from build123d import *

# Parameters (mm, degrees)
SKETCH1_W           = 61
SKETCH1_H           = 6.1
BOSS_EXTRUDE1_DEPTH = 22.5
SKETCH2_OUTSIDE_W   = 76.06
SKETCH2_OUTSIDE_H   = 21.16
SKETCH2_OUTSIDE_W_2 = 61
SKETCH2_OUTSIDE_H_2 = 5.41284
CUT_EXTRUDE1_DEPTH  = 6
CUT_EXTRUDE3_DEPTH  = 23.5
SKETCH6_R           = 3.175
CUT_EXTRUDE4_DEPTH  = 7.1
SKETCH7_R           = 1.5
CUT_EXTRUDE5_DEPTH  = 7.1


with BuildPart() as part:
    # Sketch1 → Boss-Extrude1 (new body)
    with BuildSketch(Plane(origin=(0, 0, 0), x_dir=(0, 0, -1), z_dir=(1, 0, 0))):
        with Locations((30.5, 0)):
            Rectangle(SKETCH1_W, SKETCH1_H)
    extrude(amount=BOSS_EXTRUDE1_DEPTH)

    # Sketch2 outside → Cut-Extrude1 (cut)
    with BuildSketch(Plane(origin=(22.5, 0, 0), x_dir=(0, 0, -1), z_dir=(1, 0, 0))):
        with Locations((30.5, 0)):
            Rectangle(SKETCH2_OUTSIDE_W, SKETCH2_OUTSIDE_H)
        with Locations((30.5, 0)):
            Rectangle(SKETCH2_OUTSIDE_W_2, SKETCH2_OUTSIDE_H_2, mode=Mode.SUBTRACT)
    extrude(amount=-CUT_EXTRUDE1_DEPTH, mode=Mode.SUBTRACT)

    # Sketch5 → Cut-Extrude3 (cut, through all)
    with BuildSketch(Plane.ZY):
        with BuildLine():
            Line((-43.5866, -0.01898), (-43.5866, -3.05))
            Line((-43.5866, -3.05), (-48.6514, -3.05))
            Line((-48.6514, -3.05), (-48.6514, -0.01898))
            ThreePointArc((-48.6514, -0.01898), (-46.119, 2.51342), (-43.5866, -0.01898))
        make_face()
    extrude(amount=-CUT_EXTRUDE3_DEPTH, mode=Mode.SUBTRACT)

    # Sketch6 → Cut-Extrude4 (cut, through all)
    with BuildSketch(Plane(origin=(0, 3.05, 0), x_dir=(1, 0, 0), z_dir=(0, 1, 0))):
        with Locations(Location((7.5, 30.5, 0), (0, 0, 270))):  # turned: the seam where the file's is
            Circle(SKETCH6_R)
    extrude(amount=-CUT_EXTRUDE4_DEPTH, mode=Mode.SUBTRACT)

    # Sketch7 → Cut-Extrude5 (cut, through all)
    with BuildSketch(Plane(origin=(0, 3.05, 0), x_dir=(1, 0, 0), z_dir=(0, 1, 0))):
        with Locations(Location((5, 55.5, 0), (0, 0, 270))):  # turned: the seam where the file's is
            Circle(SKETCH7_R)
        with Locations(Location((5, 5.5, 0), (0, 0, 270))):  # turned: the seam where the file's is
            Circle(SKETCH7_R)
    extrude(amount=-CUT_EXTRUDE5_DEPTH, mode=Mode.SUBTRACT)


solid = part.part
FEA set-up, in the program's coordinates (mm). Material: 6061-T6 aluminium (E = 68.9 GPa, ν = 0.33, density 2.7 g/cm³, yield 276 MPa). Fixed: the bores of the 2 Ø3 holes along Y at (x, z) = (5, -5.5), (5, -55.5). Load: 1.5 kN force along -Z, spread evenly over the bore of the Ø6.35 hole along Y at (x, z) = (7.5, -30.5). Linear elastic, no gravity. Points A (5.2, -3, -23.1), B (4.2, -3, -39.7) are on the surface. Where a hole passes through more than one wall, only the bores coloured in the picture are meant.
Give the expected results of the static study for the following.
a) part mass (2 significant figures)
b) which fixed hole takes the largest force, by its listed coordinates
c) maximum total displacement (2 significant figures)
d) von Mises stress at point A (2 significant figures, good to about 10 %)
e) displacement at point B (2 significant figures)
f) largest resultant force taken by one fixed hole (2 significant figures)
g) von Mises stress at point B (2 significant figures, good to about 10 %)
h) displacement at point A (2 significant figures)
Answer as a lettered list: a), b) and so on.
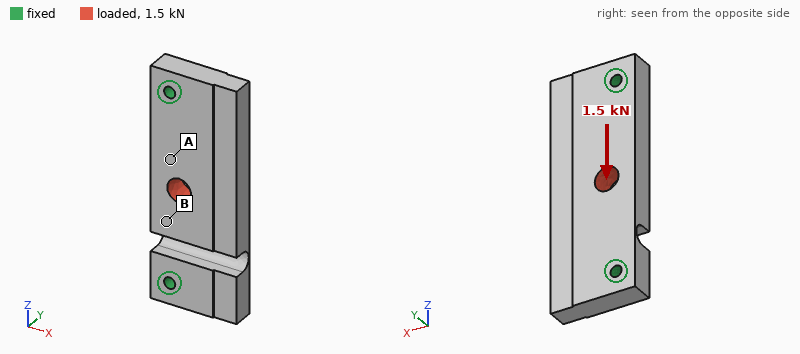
a) 20 g
b) (5, -5.5)
c) 9.3 µm
d) 17 MPa
e) 8.2 µm
f) 1.2 kN
g) 4.9 MPa
h) 4.9 µm
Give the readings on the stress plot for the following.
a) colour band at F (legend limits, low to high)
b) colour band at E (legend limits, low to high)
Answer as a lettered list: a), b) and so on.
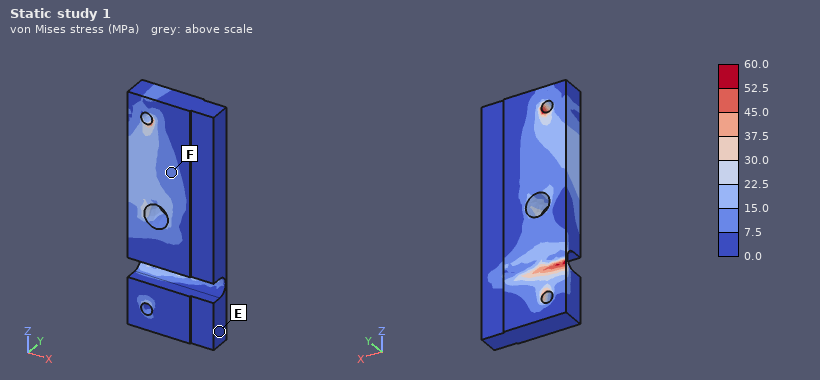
a) 7.5 to 15.0 MPa
b) 0.0 to 7.5 MPa
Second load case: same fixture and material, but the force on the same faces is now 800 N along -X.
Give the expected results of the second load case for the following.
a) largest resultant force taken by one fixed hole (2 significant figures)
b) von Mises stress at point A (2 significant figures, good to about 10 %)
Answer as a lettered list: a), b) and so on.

a) 450 N
b) 13 MPa
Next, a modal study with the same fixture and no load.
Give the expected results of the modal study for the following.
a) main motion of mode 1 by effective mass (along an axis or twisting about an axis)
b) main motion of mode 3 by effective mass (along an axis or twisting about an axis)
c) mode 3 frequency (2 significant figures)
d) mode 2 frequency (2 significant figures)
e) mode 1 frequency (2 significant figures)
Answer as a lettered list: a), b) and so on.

a) along Y
b) along X
c) 13 kHz
d) 9600 Hz
e) 6400 Hz
